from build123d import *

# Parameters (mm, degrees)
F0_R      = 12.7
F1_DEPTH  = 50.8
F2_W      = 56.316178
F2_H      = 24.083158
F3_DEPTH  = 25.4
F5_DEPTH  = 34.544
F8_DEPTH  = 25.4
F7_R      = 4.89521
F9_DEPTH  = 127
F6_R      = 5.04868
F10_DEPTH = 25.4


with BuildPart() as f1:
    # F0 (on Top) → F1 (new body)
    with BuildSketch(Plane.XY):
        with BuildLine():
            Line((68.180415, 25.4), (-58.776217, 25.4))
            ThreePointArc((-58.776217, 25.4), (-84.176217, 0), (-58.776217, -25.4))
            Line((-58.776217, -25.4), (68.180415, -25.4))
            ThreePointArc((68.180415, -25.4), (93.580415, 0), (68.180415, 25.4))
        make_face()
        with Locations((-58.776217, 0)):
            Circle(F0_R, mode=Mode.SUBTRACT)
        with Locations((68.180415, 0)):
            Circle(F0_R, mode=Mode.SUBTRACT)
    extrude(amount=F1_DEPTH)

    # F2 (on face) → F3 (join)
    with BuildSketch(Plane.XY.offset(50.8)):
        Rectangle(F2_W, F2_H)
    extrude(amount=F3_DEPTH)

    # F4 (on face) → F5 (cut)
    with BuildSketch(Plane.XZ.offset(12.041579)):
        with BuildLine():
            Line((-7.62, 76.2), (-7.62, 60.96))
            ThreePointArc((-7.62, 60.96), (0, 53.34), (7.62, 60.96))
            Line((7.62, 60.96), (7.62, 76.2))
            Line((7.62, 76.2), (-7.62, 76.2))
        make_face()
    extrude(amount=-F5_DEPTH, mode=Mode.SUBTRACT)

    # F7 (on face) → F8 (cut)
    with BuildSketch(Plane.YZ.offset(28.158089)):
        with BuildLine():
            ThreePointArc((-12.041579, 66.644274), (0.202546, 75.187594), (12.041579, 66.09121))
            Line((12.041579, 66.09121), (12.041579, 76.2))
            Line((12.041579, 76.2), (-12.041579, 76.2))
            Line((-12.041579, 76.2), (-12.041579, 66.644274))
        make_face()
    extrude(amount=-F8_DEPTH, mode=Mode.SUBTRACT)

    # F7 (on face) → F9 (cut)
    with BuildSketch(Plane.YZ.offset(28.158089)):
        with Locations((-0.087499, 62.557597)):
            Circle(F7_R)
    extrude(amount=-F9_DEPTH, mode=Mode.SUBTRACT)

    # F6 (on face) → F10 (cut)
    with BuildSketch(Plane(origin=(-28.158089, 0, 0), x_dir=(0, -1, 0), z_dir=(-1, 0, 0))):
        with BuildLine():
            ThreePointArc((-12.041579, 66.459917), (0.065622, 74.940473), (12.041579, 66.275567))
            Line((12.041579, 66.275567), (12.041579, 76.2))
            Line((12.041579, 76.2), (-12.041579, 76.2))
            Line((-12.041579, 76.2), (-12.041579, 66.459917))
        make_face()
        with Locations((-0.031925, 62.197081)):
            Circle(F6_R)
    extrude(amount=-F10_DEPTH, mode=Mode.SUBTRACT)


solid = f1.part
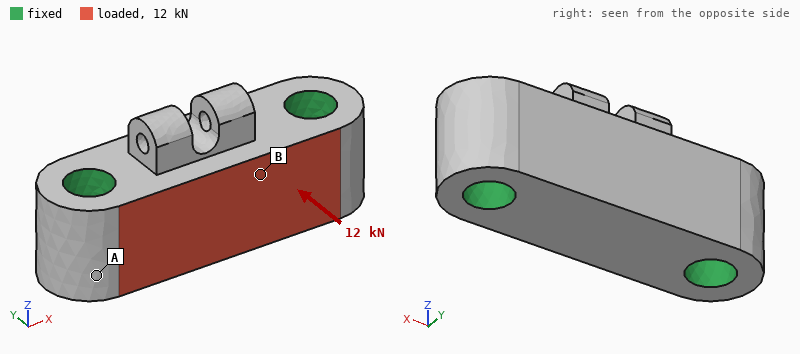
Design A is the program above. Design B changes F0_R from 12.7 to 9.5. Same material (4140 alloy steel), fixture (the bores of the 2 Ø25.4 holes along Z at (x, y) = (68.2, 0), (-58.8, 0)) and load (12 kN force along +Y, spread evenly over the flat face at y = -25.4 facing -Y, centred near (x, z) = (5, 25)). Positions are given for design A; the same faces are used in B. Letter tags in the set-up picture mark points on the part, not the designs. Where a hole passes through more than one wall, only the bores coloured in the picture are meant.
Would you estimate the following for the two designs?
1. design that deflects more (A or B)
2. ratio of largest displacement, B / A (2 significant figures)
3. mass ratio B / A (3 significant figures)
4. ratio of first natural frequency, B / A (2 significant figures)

B
1.2
1.06
0.89
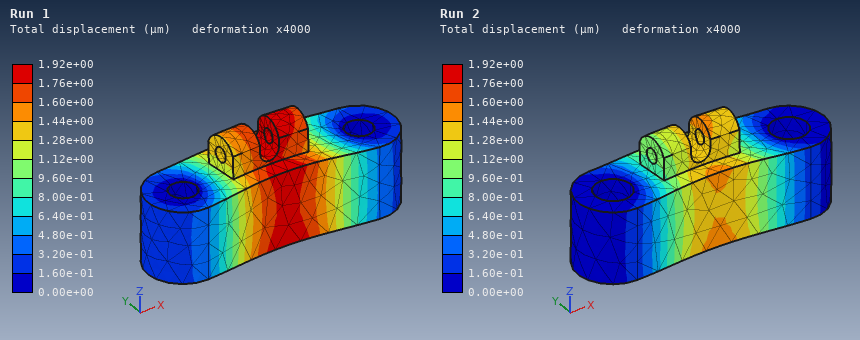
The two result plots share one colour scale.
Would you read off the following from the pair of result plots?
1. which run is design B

Run 1
